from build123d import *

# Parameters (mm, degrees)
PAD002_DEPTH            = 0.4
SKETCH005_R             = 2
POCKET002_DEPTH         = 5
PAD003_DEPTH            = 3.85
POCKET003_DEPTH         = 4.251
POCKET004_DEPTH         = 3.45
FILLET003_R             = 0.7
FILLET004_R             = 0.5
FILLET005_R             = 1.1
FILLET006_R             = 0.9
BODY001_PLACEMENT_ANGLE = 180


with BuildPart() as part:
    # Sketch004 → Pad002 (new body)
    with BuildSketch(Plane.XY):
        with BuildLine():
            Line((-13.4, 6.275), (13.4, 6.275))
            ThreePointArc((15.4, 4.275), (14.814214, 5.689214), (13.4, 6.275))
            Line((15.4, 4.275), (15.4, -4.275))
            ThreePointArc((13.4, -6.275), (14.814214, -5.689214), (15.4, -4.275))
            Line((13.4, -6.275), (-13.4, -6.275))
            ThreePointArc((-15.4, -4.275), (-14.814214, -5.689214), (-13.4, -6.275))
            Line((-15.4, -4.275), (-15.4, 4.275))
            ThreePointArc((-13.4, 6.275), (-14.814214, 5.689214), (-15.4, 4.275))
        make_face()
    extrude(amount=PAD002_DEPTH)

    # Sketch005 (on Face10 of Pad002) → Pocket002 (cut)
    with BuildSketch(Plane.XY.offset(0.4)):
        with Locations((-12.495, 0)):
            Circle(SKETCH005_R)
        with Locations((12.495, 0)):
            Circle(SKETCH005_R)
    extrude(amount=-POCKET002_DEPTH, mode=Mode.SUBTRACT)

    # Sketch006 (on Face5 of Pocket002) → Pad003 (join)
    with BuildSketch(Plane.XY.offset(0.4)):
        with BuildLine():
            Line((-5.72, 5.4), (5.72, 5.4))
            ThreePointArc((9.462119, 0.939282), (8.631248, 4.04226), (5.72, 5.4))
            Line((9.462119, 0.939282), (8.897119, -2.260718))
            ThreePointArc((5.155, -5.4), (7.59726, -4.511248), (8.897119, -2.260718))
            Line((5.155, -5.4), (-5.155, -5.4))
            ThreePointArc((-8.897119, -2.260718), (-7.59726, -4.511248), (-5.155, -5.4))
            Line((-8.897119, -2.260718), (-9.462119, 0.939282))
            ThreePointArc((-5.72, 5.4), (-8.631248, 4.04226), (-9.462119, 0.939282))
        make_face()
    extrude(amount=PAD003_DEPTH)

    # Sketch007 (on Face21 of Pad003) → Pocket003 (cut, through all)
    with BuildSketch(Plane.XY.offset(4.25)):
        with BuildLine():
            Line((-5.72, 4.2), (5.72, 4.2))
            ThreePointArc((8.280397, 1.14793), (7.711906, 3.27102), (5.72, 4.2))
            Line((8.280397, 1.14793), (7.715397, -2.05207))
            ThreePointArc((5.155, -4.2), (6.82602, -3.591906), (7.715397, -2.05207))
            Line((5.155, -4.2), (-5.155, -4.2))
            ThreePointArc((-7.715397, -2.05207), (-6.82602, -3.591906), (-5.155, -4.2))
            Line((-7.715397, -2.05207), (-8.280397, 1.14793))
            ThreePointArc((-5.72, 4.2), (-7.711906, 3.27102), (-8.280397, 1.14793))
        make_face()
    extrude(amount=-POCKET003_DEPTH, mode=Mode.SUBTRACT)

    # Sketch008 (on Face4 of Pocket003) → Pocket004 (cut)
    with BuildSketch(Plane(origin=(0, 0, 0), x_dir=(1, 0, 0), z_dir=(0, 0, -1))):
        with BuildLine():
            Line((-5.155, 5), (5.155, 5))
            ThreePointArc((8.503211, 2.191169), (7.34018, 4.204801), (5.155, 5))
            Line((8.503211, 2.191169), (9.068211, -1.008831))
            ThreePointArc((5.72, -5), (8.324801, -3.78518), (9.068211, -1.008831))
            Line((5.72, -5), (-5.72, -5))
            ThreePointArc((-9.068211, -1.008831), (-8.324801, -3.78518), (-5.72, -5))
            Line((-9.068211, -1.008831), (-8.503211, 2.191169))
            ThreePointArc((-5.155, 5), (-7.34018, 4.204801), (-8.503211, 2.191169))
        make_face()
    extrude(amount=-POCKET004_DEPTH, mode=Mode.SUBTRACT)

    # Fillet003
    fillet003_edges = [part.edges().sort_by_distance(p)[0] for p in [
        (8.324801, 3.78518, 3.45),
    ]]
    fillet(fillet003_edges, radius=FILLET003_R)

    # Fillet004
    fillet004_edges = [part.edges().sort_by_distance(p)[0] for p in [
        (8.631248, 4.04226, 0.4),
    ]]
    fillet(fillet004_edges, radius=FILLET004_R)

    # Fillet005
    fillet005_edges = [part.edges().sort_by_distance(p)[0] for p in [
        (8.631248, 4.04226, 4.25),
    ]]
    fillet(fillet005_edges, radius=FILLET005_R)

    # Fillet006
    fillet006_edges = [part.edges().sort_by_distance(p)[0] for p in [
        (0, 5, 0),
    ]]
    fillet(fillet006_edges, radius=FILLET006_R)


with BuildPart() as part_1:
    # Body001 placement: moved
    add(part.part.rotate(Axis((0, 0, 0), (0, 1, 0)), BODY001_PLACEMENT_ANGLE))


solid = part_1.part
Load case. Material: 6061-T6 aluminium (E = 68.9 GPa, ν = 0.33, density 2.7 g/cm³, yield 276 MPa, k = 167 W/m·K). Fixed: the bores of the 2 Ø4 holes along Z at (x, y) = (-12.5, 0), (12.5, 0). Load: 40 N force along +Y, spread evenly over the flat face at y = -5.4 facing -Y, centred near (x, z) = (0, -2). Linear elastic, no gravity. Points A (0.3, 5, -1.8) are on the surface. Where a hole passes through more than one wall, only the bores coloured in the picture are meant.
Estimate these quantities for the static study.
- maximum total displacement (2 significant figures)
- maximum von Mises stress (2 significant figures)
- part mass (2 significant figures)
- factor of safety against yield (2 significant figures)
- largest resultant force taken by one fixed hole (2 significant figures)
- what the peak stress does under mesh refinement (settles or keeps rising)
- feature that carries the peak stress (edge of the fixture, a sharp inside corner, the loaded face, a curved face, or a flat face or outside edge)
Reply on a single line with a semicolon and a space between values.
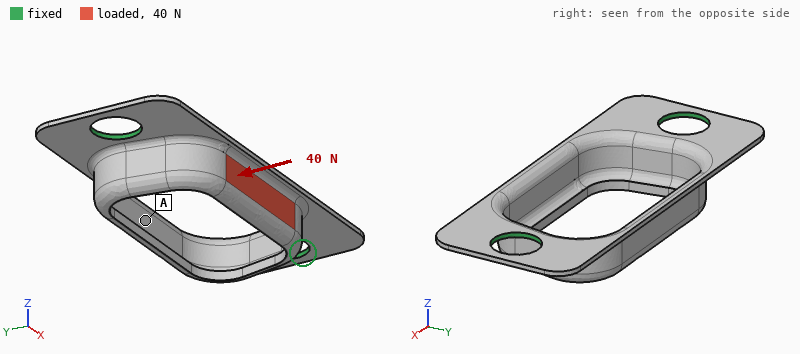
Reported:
80 µm; 170 MPa; 0.46 g; 1.6; 27 N; settles; a flat face or outside edge
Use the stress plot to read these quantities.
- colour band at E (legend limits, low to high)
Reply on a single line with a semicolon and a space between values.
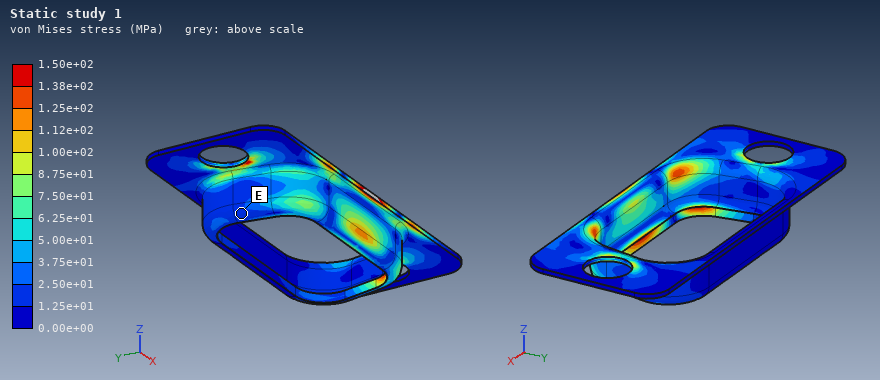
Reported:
1.25e+01 to 2.50e+01 MPa
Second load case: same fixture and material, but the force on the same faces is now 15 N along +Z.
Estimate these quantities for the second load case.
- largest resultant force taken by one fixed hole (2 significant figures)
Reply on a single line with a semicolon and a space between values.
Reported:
12 N
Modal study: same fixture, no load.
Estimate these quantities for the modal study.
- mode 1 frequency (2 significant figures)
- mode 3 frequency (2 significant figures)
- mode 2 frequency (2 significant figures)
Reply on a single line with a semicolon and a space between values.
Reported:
7100 Hz; 14 kHz; 13 kHz
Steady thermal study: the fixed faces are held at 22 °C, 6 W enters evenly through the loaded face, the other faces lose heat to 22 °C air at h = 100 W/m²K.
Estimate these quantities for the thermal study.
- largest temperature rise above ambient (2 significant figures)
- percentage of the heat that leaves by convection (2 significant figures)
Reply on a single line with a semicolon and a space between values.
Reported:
63 K; 20 %
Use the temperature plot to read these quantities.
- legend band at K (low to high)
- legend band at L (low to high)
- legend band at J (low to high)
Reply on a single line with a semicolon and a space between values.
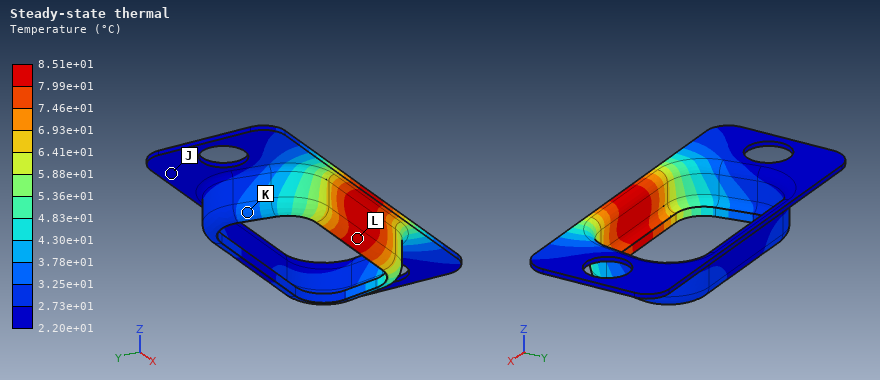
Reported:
3.25e+01 to 3.78e+01 °C; 7.99e+01 to 8.51e+01 °C; 2.20e+01 to 2.73e+01 °C
